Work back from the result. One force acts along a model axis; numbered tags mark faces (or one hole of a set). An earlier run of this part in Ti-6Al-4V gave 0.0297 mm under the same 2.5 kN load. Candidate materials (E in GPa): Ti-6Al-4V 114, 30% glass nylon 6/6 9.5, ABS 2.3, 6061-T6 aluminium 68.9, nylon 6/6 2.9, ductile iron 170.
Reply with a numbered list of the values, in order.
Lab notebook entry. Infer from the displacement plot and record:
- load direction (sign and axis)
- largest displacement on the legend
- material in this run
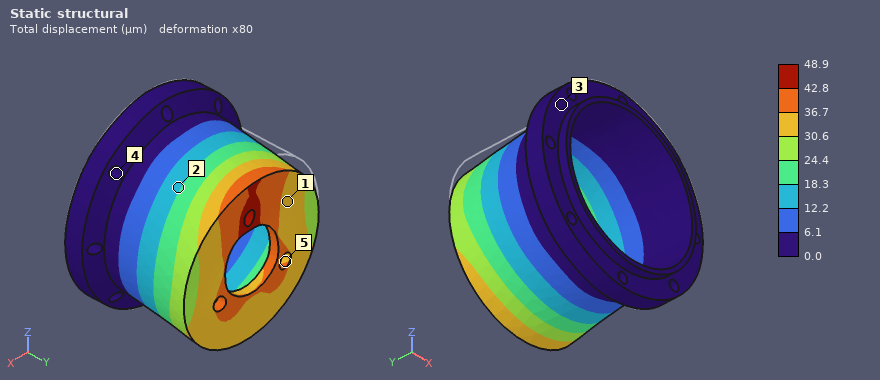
1. -Z
2. 48.9 µm
3. 6061-T6 aluminium
